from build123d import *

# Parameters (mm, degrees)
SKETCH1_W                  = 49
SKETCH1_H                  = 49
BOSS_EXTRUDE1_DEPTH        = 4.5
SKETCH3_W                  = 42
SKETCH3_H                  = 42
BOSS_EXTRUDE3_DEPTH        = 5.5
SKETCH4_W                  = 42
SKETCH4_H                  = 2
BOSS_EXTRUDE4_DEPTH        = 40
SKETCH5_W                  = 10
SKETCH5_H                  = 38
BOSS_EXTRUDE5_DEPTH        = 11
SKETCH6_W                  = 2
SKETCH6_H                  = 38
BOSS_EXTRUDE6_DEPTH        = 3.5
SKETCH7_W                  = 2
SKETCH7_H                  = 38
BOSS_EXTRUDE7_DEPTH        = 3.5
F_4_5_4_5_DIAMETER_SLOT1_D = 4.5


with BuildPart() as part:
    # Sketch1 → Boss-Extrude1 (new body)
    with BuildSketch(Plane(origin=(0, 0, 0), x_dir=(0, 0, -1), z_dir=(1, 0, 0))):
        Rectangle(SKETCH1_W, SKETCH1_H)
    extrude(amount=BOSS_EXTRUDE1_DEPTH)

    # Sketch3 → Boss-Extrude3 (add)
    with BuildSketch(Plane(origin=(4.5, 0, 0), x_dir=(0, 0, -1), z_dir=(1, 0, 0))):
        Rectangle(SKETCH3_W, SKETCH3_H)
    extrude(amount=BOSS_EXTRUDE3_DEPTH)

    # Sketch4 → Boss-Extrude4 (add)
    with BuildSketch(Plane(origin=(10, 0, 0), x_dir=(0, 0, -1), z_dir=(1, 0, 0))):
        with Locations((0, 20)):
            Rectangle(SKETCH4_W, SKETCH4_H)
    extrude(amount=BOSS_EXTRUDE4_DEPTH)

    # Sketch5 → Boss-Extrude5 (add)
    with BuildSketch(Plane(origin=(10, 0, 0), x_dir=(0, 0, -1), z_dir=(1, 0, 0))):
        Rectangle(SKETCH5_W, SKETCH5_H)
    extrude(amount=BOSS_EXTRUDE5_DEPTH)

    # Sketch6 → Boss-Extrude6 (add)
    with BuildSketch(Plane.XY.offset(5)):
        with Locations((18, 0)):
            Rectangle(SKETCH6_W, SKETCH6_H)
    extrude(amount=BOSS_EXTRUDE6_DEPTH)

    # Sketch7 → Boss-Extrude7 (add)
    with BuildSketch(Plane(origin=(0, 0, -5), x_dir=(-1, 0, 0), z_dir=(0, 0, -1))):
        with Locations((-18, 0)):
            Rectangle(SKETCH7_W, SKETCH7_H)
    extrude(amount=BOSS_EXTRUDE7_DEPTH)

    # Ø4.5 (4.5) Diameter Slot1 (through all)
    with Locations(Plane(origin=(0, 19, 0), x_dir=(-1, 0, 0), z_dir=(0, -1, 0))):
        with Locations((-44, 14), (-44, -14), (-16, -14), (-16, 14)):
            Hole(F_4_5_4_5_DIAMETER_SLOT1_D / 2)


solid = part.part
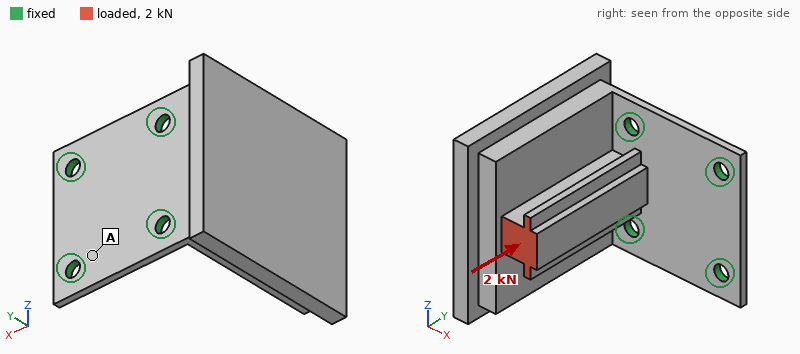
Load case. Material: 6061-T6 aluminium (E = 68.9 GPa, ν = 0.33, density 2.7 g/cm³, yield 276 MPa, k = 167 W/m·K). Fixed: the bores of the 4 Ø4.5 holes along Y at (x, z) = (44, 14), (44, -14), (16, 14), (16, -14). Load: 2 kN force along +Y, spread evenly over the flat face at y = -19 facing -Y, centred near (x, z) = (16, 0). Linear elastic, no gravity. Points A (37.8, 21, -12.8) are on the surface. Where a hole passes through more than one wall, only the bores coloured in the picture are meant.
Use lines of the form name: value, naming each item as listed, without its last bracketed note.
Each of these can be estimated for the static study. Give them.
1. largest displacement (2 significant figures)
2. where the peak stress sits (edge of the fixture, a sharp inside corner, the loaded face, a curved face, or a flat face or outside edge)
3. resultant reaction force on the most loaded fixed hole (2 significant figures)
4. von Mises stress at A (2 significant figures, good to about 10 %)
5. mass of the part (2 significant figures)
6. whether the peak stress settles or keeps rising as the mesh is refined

largest displacement: 0.11 mm
where the peak stress sits: edge of the fixture
resultant reaction force on the most loaded fixed hole: 1.0 kN
von Mises stress at A: 15 MPa
mass of the part: 77 g
whether the peak stress settles or keeps rising as the mesh is refined: keeps rising
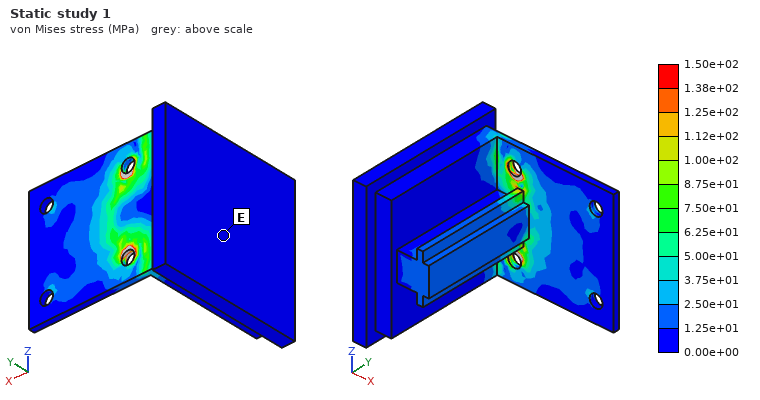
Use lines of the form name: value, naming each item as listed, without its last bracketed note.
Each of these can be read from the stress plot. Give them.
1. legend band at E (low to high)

legend band at E: 0.00e+00 to 1.25e+01 MPa
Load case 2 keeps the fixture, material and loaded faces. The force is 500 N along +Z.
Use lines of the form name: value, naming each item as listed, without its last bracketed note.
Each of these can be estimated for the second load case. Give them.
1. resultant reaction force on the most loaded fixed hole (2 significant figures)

resultant reaction force on the most loaded fixed hole: 760 N
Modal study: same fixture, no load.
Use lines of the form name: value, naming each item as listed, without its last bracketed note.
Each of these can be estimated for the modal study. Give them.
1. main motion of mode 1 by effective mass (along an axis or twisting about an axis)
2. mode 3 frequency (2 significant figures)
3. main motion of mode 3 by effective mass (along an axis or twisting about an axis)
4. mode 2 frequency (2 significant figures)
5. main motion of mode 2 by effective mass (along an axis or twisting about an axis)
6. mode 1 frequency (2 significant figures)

main motion of mode 1 by effective mass: along X
mode 3 frequency: 5700 Hz
main motion of mode 3 by effective mass: along Y
mode 2 frequency: 2600 Hz
main motion of mode 2 by effective mass: along Z
mode 1 frequency: 850 Hz
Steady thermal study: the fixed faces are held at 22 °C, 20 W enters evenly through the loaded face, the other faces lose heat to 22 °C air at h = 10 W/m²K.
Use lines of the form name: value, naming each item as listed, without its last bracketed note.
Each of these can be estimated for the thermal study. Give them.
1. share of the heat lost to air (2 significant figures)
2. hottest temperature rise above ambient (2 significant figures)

share of the heat lost to air: 5.5 %
hottest temperature rise above ambient: 25 K
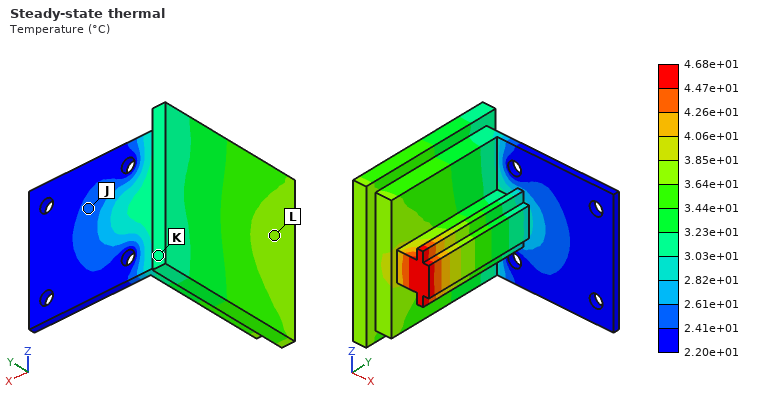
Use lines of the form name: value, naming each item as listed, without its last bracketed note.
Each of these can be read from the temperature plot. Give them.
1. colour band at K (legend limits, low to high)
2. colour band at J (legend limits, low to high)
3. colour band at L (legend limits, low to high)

colour band at K: 3.03e+01 to 3.23e+01 °C
colour band at J: 2.41e+01 to 2.61e+01 °C
colour band at L: 3.64e+01 to 3.85e+01 °C
